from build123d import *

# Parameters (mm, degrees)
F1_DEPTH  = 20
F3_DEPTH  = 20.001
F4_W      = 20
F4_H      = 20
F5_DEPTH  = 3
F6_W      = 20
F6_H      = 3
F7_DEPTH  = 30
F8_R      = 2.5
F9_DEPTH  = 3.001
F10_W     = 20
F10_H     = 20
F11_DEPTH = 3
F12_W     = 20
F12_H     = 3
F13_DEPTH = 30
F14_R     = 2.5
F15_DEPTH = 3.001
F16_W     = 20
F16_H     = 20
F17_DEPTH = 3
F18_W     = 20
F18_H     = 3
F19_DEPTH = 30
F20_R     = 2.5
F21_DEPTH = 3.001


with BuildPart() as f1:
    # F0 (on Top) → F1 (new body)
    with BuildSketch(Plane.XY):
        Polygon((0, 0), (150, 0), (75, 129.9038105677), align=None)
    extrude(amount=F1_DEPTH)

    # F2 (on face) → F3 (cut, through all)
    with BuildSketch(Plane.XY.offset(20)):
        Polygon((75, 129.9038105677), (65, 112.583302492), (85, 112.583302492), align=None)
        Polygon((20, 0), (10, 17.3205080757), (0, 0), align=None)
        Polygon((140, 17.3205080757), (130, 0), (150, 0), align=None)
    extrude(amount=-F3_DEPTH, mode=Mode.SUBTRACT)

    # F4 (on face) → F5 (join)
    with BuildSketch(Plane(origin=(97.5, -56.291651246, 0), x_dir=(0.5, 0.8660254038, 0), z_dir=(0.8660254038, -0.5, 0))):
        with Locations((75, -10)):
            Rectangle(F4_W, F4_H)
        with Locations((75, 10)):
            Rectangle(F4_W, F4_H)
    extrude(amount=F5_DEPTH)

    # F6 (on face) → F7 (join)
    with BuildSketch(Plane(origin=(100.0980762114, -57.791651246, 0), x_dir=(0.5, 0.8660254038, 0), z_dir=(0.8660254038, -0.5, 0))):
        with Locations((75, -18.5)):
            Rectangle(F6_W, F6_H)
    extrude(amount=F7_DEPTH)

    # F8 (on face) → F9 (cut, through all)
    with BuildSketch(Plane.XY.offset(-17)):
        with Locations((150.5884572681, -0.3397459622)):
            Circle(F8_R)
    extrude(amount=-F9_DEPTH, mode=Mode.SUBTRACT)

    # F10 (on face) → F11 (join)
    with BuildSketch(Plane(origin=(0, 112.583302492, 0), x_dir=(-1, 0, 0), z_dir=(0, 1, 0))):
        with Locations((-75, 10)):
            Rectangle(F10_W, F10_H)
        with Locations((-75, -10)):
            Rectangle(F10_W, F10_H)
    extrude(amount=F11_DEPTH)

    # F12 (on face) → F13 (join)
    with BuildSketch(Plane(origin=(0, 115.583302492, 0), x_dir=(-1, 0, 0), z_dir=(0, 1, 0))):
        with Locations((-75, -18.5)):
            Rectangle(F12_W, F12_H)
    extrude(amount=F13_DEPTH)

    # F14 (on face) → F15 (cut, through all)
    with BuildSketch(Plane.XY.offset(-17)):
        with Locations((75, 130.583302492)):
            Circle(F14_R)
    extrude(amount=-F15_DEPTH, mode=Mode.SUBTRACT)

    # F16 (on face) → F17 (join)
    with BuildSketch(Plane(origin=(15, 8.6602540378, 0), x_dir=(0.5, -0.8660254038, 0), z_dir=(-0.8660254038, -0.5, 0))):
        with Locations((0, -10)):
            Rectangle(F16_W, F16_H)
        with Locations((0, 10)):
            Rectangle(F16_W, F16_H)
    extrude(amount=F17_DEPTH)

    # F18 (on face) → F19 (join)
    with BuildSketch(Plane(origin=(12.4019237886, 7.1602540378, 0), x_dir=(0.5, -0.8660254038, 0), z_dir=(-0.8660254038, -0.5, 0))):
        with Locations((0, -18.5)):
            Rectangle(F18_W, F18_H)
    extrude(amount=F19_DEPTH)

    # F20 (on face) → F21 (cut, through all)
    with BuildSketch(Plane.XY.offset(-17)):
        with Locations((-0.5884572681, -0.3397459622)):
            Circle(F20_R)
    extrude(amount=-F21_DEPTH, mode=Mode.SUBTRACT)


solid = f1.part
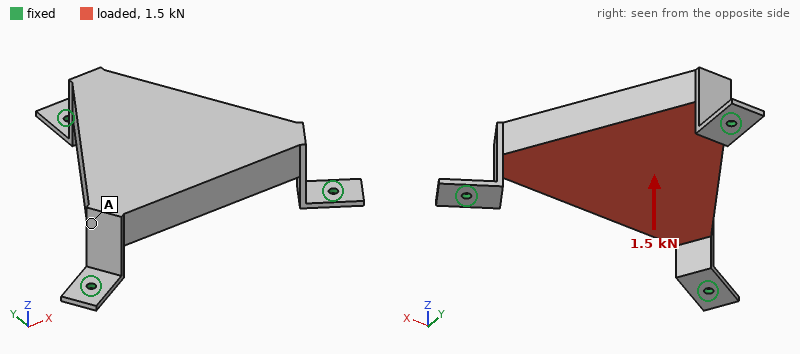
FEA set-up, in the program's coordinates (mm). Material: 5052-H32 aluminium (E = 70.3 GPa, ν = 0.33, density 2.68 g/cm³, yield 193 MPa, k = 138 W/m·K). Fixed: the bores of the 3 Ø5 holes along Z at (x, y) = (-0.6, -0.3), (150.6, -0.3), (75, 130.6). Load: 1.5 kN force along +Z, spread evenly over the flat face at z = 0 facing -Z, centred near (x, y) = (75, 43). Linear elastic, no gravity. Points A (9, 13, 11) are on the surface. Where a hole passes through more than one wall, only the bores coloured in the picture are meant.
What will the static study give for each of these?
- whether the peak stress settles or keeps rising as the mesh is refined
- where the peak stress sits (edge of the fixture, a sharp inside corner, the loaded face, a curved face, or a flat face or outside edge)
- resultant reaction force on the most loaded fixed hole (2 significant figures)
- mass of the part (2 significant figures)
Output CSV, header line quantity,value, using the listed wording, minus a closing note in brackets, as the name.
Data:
quantity,value
whether the peak stress settles or keeps rising as the mesh is refined,keeps rising
where the peak stress sits,edge of the fixture
resultant reaction force on the most loaded fixed hole,560 N
mass of the part,530 g
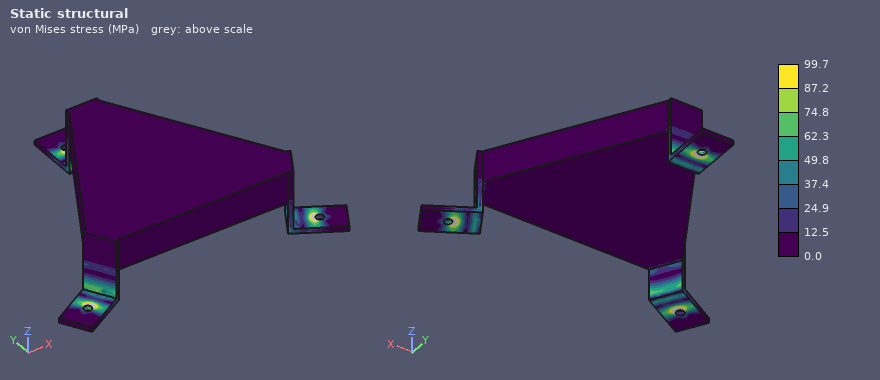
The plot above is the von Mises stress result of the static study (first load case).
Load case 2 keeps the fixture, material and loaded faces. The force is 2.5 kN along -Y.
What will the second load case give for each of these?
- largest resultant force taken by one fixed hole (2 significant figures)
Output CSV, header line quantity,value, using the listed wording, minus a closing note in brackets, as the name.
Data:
quantity,value
largest resultant force taken by one fixed hole,1.1 kN
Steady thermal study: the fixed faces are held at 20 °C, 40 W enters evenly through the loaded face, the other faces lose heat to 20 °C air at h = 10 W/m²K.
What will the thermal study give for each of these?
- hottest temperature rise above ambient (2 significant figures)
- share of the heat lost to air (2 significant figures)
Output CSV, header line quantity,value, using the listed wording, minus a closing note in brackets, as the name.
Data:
quantity,value
hottest temperature rise above ambient,50 K
share of the heat lost to air,24 %
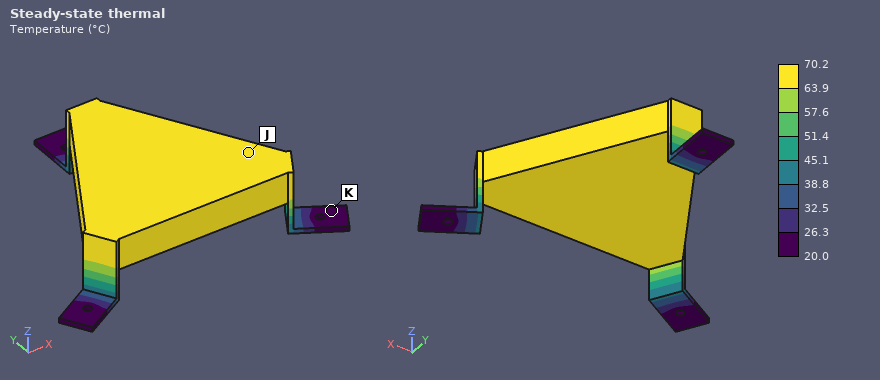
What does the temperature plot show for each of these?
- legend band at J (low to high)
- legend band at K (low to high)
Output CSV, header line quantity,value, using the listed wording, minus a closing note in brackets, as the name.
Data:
quantity,value
legend band at J,63.9 to 70.2 °C
legend band at K,20.0 to 26.3 °C
